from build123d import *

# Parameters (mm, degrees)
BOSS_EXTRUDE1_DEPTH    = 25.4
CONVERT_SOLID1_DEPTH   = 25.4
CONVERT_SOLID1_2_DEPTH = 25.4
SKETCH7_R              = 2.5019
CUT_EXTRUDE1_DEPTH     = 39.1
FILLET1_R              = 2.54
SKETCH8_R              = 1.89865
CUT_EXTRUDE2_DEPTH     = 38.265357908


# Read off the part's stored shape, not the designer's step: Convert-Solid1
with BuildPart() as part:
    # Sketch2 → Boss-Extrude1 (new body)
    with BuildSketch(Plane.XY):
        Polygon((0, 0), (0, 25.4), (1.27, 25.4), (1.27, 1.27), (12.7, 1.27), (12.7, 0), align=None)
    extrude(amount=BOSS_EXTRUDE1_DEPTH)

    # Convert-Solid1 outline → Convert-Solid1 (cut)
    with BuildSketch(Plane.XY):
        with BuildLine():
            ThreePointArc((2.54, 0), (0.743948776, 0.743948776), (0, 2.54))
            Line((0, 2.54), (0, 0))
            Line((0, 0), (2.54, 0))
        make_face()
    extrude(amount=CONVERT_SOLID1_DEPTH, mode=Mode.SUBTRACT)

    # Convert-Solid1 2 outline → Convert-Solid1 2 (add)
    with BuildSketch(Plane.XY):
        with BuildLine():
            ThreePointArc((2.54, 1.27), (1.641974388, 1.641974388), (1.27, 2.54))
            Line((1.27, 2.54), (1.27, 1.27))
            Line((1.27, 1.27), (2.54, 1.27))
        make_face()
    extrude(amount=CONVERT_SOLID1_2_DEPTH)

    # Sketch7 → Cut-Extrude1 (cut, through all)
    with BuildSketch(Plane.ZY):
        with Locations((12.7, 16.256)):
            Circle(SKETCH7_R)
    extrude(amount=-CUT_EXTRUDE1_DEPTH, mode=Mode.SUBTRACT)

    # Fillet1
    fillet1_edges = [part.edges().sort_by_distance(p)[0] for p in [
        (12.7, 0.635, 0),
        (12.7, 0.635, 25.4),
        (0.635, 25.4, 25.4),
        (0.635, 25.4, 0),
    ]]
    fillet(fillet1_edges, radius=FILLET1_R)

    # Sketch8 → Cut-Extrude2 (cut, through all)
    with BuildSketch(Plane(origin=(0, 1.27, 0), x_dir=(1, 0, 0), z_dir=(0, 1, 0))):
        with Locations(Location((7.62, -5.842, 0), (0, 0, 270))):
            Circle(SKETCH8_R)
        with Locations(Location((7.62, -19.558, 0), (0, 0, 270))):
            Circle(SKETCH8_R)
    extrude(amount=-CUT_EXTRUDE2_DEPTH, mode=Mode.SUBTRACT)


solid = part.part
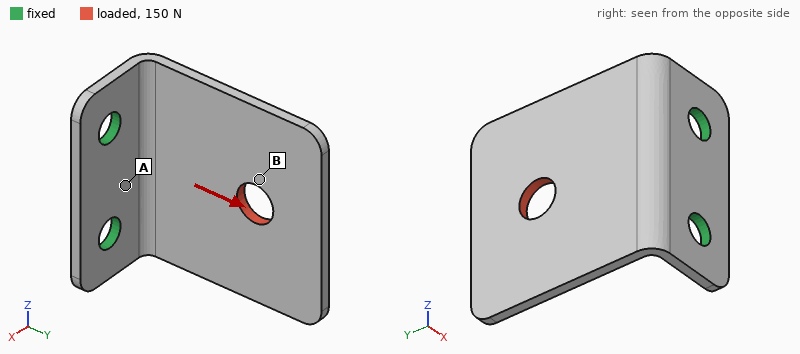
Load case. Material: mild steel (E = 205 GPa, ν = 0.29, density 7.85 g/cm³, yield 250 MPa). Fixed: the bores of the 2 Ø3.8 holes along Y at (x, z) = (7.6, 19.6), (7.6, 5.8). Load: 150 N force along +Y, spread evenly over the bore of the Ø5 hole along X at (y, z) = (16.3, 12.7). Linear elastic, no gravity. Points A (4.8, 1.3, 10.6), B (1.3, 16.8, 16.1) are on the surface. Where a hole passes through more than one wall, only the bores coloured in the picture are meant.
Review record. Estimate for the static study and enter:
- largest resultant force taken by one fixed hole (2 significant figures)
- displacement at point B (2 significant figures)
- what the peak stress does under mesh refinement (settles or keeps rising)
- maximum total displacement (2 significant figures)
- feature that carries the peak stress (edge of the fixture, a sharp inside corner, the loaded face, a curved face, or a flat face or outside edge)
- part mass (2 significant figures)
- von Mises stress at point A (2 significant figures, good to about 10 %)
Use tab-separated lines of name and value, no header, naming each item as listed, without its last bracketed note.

largest resultant force taken by one fixed hole	75 N
displacement at point B	48 µm
what the peak stress does under mesh refinement	keeps rising
maximum total displacement	74 µm
feature that carries the peak stress	edge of the fixture
part mass	8.6 g
von Mises stress at point A	59 MPa
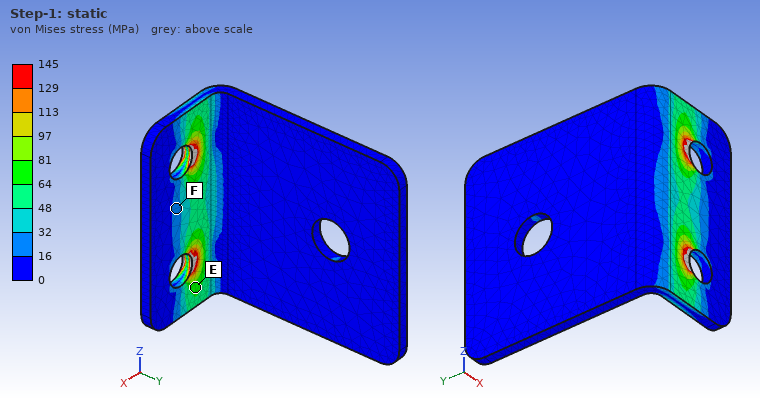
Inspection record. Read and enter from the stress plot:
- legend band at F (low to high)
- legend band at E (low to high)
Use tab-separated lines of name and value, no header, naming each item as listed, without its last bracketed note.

legend band at F	16 to 32 MPa
legend band at E	64 to 81 MPa
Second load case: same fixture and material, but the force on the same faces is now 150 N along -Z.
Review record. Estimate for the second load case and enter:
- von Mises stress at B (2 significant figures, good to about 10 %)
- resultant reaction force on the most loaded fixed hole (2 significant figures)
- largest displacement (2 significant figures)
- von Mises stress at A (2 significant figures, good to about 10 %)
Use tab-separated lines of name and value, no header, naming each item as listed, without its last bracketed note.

von Mises stress at B	16 MPa
resultant reaction force on the most loaded fixed hole	170 N
largest displacement	62 µm
von Mises stress at A	59 MPa
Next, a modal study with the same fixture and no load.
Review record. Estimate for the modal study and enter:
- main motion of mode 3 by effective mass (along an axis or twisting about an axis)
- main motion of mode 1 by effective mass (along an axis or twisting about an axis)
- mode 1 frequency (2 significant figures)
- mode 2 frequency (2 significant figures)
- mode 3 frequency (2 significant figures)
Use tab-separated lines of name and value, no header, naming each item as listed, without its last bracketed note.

main motion of mode 3 by effective mass	along Z
main motion of mode 1 by effective mass	along X
mode 1 frequency	1300 Hz
mode 2 frequency	3400 Hz
mode 3 frequency	5100 Hz
